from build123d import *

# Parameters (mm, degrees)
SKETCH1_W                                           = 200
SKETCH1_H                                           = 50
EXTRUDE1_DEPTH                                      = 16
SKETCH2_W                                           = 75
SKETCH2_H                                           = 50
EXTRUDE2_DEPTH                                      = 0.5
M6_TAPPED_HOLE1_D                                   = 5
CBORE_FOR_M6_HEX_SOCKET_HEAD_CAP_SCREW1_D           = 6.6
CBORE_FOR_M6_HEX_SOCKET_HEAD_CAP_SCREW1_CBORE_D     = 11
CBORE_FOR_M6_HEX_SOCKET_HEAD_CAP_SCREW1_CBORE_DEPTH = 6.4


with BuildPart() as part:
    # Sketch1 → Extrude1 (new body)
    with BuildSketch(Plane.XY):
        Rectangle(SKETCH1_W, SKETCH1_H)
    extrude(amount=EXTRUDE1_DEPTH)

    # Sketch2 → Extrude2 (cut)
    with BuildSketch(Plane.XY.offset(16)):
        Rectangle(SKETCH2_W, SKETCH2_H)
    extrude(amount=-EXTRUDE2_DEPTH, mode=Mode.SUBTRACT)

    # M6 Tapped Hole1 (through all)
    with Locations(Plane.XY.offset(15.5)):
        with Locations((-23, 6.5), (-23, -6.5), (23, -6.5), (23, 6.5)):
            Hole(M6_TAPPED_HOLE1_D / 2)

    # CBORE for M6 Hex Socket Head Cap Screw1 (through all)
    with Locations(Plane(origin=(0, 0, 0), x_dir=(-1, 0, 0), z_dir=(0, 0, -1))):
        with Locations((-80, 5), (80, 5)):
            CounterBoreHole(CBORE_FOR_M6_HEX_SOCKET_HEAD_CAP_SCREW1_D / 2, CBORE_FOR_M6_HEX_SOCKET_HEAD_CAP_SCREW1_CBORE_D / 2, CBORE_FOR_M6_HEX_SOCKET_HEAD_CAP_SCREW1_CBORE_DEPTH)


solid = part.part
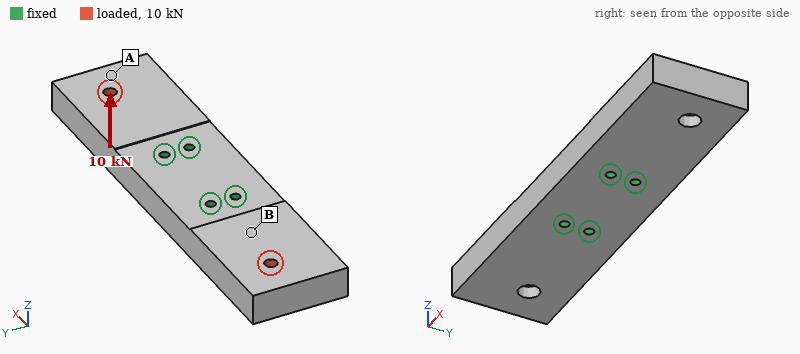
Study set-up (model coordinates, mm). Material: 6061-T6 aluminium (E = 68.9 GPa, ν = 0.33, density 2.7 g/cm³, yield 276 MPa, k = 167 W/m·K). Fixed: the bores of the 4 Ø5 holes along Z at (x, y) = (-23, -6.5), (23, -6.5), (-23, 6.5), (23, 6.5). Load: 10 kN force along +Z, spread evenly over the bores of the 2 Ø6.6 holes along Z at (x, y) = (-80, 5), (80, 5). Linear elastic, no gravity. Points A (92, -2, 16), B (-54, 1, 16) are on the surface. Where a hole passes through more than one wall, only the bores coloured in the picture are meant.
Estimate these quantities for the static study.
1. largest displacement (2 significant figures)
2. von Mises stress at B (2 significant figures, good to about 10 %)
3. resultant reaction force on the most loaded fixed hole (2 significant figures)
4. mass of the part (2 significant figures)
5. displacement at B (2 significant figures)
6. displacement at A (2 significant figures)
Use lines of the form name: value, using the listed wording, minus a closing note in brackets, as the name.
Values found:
largest displacement: 0.50 mm
von Mises stress at B: 62 MPa
resultant reaction force on the most loaded fixed hole: 3.3 kN
mass of the part: 420 g
displacement at B: 0.14 mm
displacement at A: 0.42 mm
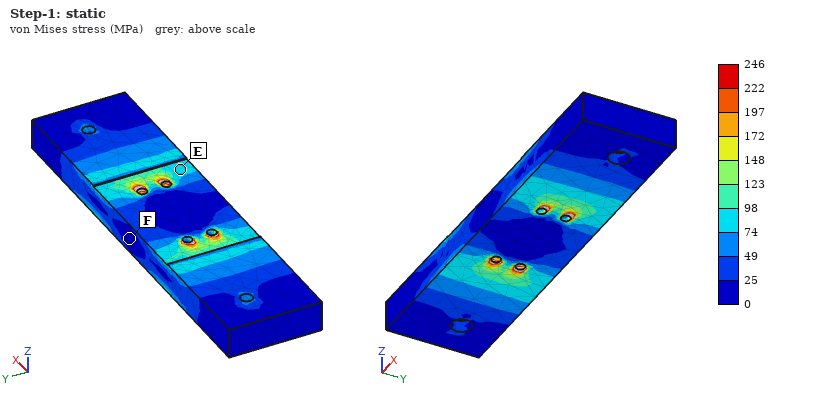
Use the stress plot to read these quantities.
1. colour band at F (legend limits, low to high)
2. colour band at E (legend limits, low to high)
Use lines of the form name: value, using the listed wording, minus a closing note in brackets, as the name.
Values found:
colour band at F: 0 to 25 MPa
colour band at E: 74 to 98 MPa
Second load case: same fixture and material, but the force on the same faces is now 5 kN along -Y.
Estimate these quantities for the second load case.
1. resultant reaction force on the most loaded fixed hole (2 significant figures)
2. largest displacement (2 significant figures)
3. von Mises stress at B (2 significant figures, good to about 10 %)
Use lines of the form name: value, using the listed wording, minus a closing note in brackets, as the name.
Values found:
resultant reaction force on the most loaded fixed hole: 3.2 kN
largest displacement: 49 µm
von Mises stress at B: 12 MPa
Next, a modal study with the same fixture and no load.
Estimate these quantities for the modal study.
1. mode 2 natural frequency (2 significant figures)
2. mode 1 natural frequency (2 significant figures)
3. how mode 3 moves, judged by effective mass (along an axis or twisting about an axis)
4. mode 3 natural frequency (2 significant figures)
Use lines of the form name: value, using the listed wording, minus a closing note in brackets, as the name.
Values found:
mode 2 natural frequency: 2000 Hz
mode 1 natural frequency: 2000 Hz
how mode 3 moves, judged by effective mass: twisting about Z
mode 3 natural frequency: 4100 Hz
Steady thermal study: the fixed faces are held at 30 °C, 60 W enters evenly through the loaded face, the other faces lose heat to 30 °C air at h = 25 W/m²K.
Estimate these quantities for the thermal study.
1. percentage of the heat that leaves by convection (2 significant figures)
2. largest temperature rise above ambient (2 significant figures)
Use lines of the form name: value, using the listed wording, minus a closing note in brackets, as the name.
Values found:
percentage of the heat that leaves by convection: 8.1 %
largest temperature rise above ambient: 17 K
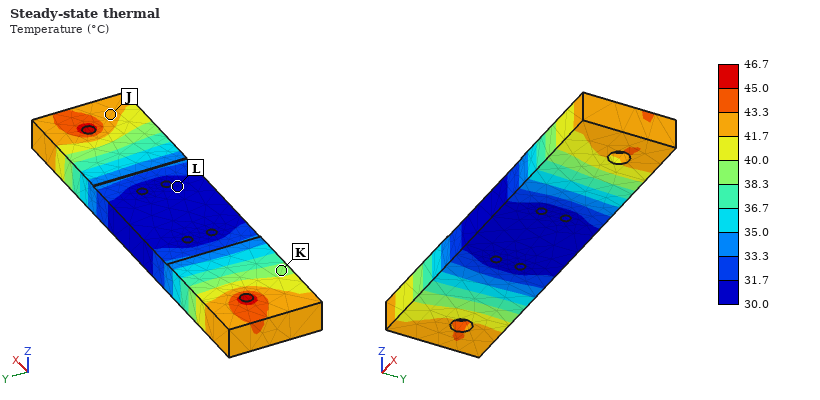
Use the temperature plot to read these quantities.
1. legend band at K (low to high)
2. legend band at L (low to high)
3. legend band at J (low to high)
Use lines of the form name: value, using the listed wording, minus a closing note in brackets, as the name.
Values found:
legend band at K: 38.3 to 40.0 °C
legend band at L: 30.0 to 31.7 °C
legend band at J: 41.7 to 43.3 °C
